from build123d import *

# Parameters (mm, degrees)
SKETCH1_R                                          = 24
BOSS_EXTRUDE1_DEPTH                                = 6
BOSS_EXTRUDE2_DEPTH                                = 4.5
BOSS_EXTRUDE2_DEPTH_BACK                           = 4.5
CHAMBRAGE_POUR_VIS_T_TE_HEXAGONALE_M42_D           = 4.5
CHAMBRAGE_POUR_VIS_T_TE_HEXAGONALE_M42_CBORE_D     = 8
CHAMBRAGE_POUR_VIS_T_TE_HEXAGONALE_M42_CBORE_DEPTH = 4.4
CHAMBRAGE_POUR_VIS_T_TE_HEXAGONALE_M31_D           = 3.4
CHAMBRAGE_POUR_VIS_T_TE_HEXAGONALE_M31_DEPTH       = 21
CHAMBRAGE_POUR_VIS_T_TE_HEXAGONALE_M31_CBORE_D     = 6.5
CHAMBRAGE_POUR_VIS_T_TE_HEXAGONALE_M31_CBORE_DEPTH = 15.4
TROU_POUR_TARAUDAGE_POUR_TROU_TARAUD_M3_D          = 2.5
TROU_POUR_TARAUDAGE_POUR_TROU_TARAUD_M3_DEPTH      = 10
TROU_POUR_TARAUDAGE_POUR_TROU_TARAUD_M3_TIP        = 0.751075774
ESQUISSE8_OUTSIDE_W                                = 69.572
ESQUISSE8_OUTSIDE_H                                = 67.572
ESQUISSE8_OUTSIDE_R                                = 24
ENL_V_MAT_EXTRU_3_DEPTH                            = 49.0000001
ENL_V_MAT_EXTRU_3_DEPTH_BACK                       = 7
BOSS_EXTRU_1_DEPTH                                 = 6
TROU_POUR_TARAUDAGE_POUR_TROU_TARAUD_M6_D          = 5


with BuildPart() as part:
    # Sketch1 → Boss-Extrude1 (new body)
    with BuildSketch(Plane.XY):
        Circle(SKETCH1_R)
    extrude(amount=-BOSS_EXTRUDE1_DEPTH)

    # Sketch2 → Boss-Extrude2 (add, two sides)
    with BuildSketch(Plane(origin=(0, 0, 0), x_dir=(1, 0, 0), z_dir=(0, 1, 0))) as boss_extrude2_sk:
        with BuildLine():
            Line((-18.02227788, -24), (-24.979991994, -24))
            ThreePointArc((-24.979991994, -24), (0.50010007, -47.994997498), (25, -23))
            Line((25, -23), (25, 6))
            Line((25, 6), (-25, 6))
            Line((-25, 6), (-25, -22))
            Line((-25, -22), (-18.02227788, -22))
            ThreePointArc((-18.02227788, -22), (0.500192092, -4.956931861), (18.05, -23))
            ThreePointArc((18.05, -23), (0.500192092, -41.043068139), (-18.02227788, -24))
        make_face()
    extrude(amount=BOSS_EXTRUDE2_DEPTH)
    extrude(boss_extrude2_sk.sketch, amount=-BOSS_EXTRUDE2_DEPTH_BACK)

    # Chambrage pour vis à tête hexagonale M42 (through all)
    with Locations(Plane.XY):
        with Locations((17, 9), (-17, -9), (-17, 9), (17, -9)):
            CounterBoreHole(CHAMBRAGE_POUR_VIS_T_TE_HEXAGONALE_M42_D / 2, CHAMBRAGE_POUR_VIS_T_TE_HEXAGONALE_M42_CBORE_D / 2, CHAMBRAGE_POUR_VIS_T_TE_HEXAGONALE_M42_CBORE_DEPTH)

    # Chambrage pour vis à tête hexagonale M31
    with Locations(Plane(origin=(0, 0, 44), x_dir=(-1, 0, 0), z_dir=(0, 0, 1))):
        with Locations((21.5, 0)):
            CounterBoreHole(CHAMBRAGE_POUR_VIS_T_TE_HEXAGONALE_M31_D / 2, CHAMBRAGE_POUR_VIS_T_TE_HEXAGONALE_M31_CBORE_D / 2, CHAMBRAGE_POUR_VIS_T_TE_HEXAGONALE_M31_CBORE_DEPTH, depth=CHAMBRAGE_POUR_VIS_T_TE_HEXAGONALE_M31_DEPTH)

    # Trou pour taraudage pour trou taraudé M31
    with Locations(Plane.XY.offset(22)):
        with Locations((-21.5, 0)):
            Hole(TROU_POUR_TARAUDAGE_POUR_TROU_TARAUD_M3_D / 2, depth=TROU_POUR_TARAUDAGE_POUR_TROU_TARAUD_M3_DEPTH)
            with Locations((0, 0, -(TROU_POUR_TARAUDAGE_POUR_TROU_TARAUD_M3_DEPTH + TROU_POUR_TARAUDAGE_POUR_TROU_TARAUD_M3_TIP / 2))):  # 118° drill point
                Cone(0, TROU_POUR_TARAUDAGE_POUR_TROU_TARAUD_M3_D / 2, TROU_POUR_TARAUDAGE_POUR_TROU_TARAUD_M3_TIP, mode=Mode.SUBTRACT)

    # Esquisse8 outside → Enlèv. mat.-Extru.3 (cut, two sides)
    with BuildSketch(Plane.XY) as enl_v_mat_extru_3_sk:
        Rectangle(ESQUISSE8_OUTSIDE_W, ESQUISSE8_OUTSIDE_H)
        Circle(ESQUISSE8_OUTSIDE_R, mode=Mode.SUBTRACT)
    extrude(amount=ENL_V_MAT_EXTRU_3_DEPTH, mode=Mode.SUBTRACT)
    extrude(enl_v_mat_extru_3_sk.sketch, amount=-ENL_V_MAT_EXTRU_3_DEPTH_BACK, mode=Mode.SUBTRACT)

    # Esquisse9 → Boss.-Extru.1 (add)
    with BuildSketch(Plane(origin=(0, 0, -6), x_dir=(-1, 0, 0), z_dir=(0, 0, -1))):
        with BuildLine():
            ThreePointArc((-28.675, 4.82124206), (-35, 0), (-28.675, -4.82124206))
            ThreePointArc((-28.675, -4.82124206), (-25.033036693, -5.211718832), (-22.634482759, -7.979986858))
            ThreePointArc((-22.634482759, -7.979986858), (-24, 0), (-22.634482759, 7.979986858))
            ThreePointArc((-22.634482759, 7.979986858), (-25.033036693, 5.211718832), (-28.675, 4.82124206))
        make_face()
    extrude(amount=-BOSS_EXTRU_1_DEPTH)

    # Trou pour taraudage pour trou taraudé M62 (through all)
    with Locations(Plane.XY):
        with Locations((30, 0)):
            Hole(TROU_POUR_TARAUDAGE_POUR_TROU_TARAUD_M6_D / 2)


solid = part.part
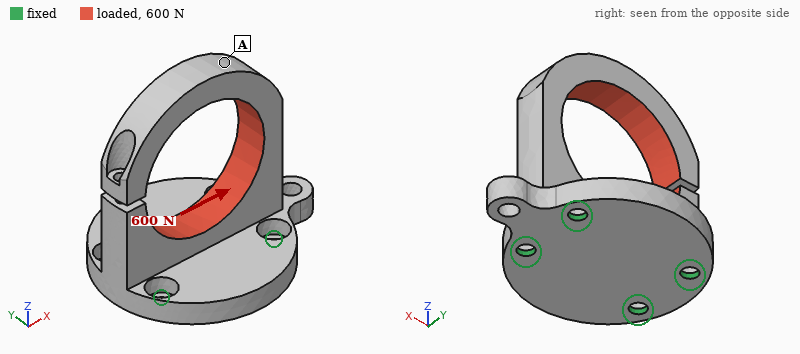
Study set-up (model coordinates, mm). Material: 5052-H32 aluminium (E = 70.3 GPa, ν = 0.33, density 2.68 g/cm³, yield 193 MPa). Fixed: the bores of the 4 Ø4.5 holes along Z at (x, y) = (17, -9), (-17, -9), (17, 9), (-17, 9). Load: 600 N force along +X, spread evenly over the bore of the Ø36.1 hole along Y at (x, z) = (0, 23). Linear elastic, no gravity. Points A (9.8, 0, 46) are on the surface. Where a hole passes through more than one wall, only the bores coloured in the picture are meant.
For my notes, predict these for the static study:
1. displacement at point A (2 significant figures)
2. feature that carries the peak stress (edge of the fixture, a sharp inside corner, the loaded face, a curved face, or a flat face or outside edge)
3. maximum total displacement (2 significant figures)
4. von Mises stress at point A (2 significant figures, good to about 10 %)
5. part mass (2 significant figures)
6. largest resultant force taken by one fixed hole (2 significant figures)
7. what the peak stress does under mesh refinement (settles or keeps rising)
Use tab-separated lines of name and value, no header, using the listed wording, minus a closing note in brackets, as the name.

displacement at point A	0.22 mm
feature that carries the peak stress	edge of the fixture
maximum total displacement	0.29 mm
von Mises stress at point A	13 MPa
part mass	52 g
largest resultant force taken by one fixed hole	420 N
what the peak stress does under mesh refinement	keeps rising
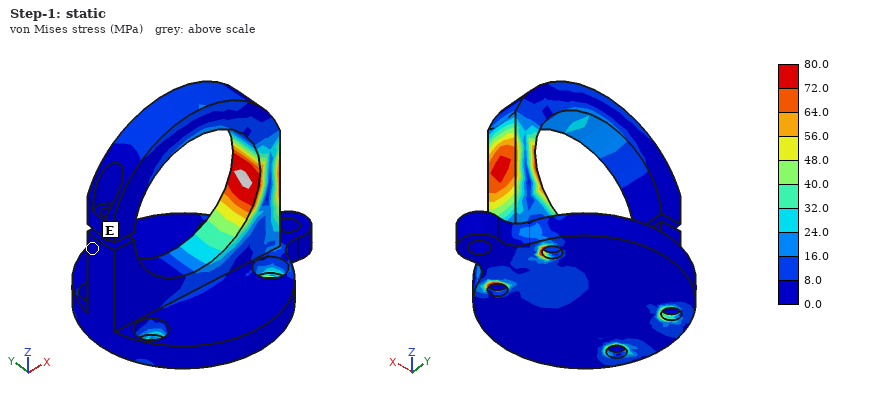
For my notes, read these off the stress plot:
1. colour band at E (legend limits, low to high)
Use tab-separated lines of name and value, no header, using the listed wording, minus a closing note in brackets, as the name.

colour band at E	0.0 to 8.0 MPa
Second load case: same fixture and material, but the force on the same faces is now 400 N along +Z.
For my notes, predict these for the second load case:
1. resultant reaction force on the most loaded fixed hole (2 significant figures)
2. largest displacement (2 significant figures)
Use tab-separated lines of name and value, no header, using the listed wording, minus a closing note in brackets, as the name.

resultant reaction force on the most loaded fixed hole	140 N
largest displacement	0.42 mm
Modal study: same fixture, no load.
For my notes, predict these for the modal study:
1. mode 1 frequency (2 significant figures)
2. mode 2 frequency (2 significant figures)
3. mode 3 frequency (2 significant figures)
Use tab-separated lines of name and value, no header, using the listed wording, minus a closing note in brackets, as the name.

mode 1 frequency	1200 Hz
mode 2 frequency	1200 Hz
mode 3 frequency	3100 Hz
